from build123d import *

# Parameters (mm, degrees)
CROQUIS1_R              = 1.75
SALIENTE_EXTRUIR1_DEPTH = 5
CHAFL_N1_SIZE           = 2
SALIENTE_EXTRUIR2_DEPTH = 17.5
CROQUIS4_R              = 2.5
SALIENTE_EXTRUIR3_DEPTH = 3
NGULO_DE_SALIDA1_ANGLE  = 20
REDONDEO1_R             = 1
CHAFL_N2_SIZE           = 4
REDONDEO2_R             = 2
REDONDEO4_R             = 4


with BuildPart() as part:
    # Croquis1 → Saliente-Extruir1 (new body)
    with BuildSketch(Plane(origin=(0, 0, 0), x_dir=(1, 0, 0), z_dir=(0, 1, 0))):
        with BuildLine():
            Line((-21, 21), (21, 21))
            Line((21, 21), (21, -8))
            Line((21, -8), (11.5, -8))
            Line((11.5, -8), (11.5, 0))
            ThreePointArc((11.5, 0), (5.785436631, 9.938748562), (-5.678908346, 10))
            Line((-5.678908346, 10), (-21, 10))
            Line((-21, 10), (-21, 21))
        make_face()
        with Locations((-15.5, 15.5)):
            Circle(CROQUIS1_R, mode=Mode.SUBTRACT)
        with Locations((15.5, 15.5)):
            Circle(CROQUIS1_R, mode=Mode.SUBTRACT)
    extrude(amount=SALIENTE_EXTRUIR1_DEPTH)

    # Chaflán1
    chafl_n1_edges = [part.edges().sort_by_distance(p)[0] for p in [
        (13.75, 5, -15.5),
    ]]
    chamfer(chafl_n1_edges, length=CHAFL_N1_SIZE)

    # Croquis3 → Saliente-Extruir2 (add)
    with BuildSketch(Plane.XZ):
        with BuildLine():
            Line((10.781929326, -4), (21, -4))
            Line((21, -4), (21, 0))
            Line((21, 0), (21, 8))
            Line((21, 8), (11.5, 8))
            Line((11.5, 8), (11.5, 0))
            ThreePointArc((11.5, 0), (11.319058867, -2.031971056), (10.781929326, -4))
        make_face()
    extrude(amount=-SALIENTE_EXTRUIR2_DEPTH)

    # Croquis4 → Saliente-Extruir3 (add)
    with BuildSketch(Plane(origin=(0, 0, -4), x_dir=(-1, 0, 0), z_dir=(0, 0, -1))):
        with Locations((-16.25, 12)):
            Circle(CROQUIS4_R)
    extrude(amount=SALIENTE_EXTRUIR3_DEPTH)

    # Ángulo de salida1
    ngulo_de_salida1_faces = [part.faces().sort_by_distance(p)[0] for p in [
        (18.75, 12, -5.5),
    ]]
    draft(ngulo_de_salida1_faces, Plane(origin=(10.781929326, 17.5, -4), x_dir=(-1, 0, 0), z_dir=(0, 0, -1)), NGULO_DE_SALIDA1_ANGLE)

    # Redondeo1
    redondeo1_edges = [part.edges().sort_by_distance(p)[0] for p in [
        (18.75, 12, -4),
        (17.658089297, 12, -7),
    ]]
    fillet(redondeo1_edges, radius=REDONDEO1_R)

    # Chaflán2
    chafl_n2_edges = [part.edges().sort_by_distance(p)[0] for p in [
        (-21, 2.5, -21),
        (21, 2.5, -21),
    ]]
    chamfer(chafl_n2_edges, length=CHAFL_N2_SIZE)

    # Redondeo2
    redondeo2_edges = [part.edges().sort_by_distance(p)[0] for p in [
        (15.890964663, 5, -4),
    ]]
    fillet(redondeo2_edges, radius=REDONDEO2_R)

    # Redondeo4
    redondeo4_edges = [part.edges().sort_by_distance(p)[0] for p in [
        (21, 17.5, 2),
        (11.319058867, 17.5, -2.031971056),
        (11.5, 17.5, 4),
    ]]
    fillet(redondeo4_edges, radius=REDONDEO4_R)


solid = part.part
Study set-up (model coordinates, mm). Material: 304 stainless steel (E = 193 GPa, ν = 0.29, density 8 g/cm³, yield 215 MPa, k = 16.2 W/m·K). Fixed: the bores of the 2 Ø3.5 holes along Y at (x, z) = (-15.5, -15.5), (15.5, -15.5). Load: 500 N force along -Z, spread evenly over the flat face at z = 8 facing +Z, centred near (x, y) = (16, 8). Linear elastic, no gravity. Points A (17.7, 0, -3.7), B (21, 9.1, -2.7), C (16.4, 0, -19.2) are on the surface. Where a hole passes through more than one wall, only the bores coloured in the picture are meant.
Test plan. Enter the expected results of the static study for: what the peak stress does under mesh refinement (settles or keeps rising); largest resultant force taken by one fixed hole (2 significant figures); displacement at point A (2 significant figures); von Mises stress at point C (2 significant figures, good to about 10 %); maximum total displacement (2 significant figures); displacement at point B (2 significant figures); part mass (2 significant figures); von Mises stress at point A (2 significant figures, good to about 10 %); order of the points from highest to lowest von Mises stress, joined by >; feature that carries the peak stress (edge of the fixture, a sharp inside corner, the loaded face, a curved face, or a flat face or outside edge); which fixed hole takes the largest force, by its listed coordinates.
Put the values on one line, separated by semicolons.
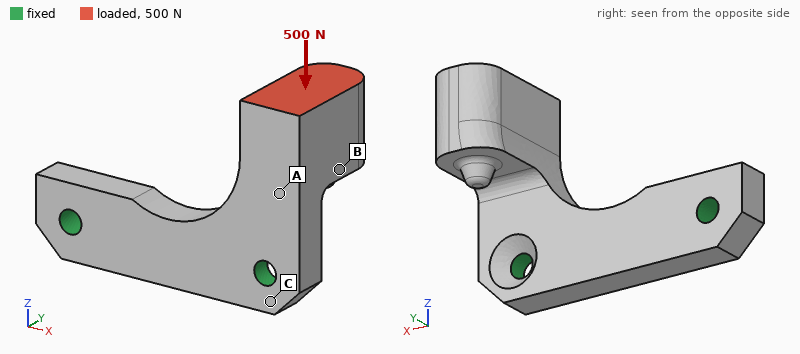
keeps rising; 490 N; 13 µm; 19 MPa; 47 µm; 20 µm; 35 g; 37 MPa; A > C > B; edge of the fixture; (15.5, -15.5)
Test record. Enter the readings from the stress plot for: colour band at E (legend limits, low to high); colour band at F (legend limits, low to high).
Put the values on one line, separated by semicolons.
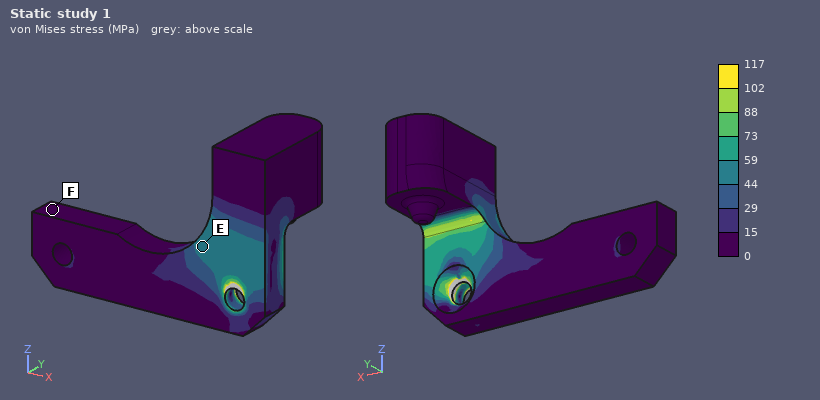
44 to 59 MPa; 0 to 15 MPa
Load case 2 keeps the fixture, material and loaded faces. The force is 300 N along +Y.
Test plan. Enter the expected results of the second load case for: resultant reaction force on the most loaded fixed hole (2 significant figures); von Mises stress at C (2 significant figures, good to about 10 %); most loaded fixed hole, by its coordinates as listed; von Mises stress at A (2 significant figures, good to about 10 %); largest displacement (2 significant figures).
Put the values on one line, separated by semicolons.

330 N; 25 MPa; (15.5, -15.5); 59 MPa; 83 µm
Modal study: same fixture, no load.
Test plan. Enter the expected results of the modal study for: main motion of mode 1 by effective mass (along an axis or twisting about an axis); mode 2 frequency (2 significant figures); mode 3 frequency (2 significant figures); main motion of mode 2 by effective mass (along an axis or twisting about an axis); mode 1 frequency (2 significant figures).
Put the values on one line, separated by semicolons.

along Y; 6100 Hz; 13 kHz; along X; 3300 Hz
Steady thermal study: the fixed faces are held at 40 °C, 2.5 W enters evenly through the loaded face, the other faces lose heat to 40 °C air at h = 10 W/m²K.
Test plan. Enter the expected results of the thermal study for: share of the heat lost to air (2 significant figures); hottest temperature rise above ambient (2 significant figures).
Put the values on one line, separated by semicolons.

14 %; 46 K
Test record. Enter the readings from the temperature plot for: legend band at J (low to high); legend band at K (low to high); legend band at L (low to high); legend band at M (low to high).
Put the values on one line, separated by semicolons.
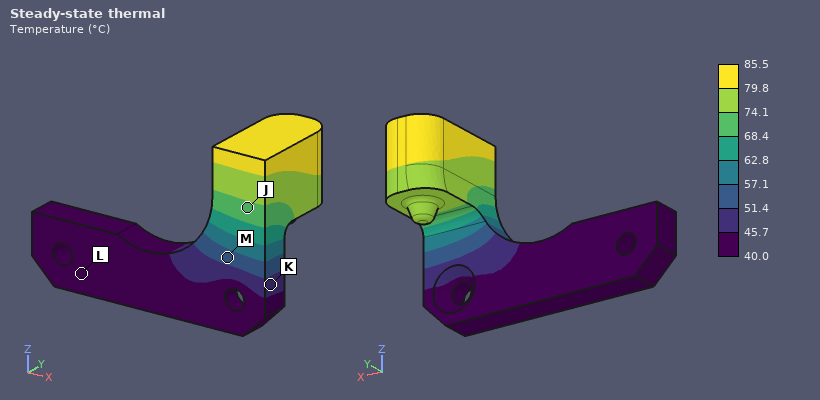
68.4 to 74.1 °C; 45.7 to 51.4 °C; 40.0 to 45.7 °C; 51.4 to 57.1 °C
